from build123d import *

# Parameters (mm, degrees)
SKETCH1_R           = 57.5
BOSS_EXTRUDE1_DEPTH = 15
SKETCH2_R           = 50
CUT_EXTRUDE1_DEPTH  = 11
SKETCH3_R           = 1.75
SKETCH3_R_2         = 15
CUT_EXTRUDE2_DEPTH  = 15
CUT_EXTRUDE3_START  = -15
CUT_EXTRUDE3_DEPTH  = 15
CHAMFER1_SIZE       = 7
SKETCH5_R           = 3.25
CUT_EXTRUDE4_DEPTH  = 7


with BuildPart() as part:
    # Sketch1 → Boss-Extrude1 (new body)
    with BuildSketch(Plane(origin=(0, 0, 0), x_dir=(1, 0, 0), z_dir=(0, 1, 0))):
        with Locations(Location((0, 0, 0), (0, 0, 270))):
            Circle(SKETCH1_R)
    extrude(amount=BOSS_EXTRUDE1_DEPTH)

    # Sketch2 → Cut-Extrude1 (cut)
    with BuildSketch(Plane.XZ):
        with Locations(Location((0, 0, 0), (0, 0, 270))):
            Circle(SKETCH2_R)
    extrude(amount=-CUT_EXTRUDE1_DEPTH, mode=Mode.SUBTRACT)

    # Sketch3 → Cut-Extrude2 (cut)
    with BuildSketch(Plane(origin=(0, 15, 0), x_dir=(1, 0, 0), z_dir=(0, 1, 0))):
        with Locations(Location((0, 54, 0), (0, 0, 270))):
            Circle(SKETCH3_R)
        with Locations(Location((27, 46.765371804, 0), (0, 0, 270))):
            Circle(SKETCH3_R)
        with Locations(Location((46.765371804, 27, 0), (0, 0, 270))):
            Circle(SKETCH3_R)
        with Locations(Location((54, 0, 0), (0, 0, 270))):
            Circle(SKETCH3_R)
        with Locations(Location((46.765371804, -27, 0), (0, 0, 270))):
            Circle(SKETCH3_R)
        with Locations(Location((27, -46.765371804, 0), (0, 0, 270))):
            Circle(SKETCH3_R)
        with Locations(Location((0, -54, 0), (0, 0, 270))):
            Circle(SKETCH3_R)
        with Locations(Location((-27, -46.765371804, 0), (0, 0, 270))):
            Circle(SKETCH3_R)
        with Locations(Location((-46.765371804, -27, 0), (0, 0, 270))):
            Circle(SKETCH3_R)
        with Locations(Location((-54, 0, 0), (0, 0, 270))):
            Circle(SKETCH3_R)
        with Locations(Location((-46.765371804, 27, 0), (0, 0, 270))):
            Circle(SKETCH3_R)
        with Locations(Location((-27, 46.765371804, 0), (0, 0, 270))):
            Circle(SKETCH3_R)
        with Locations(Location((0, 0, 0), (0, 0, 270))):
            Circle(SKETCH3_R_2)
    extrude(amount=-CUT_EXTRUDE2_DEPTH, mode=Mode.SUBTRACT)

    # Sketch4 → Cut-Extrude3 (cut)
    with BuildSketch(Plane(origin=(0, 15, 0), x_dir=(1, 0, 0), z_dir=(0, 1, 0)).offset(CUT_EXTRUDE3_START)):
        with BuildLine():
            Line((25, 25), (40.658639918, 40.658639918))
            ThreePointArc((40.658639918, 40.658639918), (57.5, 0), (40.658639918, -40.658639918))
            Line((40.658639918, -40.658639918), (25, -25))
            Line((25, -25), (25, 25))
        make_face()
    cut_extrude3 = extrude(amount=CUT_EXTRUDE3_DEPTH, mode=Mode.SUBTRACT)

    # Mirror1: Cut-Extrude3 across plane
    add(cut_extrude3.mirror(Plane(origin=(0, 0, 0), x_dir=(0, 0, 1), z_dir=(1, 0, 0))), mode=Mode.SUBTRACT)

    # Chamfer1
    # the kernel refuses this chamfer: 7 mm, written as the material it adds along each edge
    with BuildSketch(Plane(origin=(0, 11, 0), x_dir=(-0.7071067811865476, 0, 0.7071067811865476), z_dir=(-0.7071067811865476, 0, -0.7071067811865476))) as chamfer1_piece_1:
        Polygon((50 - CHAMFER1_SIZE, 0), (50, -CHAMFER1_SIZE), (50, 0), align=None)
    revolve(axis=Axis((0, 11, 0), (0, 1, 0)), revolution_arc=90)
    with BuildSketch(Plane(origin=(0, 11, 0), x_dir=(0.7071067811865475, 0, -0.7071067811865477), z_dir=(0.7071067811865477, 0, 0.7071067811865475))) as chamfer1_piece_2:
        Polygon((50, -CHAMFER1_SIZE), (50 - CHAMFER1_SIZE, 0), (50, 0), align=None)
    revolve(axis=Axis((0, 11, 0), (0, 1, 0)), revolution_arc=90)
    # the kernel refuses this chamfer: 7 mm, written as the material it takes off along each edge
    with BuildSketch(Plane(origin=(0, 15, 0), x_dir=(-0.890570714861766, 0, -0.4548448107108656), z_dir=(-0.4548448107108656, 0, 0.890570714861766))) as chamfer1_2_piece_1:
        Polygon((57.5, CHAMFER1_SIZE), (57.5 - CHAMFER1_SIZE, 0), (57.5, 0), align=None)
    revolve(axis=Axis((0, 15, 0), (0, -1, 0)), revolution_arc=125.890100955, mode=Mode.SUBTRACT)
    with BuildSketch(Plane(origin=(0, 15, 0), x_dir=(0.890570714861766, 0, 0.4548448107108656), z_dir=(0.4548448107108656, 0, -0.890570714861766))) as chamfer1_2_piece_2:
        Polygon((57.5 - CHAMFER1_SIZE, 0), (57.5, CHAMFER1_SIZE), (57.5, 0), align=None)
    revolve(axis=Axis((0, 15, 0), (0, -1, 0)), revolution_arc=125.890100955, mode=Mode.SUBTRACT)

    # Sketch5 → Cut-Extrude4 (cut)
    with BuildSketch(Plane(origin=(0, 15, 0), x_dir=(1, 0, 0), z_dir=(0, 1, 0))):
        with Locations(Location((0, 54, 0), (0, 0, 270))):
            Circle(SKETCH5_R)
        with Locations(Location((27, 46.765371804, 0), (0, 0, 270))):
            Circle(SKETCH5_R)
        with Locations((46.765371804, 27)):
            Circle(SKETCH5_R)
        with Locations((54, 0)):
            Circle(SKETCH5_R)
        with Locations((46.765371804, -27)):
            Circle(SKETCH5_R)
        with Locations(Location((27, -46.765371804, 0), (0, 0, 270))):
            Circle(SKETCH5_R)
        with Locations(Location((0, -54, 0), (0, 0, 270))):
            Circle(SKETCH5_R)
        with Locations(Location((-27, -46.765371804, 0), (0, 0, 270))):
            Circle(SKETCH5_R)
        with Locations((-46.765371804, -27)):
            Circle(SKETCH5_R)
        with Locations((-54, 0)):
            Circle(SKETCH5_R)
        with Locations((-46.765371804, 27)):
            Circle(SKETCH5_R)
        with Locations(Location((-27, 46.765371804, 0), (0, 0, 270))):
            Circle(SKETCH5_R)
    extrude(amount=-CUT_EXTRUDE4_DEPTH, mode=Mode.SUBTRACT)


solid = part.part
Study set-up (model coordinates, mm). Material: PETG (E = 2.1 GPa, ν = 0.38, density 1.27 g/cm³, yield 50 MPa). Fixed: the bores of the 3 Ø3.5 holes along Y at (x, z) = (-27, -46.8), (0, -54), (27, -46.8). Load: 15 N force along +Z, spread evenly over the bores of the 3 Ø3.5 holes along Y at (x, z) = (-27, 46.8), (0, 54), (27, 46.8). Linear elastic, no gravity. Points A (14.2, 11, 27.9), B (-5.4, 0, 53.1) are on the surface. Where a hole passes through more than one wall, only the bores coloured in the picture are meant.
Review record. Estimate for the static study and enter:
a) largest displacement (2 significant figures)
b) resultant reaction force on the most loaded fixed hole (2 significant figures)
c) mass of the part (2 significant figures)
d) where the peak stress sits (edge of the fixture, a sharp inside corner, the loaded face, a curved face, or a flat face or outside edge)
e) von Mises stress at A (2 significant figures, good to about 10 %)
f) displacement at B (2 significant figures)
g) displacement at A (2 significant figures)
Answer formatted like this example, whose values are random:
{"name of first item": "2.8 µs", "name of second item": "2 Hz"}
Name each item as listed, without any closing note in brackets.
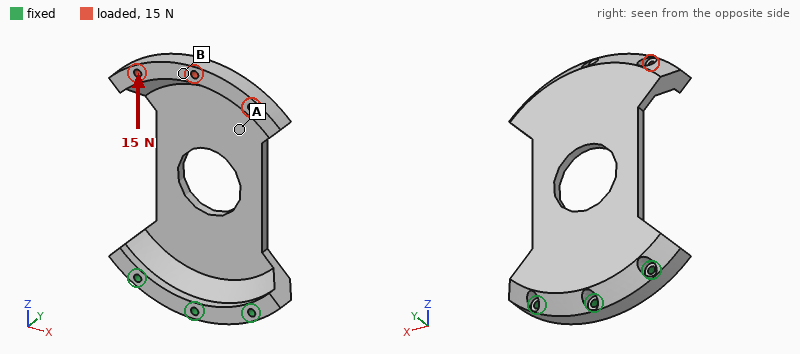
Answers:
{"largest displacement": "1.6 mm", "resultant reaction force on the most loaded fixed hole": "6.0 N", "mass of the part": "45 g", "where the peak stress sits": "a curved face", "von Mises stress at A": "0.93 MPa", "displacement at B": "1.5 mm", "displacement at A": "0.77 mm"}
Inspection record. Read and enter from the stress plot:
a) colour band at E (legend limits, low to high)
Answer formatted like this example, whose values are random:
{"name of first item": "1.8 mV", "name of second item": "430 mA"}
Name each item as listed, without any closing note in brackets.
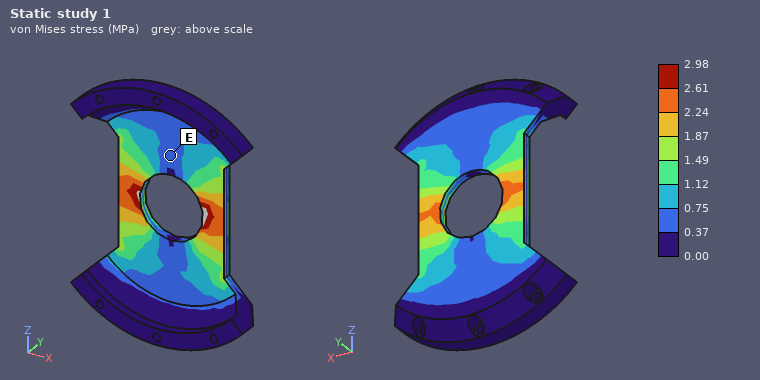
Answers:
{"colour band at E": "0.37 to 0.75 MPa"}
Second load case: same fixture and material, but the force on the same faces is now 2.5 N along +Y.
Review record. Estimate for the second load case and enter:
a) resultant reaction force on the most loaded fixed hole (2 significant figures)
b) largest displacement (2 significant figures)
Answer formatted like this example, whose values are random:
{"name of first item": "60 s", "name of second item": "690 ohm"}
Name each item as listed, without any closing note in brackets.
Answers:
{"resultant reaction force on the most loaded fixed hole": "7.2 N", "largest displacement": "1.7 mm"}
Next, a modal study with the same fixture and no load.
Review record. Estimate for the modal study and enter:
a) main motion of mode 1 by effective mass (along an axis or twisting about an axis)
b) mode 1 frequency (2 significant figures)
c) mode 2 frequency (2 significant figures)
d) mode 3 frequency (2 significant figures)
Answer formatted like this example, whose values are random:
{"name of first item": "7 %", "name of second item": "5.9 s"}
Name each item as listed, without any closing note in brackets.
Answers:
{"main motion of mode 1 by effective mass": "along Y", "mode 1 frequency": "53 Hz", "mode 2 frequency": "180 Hz", "mode 3 frequency": "450 Hz"}
